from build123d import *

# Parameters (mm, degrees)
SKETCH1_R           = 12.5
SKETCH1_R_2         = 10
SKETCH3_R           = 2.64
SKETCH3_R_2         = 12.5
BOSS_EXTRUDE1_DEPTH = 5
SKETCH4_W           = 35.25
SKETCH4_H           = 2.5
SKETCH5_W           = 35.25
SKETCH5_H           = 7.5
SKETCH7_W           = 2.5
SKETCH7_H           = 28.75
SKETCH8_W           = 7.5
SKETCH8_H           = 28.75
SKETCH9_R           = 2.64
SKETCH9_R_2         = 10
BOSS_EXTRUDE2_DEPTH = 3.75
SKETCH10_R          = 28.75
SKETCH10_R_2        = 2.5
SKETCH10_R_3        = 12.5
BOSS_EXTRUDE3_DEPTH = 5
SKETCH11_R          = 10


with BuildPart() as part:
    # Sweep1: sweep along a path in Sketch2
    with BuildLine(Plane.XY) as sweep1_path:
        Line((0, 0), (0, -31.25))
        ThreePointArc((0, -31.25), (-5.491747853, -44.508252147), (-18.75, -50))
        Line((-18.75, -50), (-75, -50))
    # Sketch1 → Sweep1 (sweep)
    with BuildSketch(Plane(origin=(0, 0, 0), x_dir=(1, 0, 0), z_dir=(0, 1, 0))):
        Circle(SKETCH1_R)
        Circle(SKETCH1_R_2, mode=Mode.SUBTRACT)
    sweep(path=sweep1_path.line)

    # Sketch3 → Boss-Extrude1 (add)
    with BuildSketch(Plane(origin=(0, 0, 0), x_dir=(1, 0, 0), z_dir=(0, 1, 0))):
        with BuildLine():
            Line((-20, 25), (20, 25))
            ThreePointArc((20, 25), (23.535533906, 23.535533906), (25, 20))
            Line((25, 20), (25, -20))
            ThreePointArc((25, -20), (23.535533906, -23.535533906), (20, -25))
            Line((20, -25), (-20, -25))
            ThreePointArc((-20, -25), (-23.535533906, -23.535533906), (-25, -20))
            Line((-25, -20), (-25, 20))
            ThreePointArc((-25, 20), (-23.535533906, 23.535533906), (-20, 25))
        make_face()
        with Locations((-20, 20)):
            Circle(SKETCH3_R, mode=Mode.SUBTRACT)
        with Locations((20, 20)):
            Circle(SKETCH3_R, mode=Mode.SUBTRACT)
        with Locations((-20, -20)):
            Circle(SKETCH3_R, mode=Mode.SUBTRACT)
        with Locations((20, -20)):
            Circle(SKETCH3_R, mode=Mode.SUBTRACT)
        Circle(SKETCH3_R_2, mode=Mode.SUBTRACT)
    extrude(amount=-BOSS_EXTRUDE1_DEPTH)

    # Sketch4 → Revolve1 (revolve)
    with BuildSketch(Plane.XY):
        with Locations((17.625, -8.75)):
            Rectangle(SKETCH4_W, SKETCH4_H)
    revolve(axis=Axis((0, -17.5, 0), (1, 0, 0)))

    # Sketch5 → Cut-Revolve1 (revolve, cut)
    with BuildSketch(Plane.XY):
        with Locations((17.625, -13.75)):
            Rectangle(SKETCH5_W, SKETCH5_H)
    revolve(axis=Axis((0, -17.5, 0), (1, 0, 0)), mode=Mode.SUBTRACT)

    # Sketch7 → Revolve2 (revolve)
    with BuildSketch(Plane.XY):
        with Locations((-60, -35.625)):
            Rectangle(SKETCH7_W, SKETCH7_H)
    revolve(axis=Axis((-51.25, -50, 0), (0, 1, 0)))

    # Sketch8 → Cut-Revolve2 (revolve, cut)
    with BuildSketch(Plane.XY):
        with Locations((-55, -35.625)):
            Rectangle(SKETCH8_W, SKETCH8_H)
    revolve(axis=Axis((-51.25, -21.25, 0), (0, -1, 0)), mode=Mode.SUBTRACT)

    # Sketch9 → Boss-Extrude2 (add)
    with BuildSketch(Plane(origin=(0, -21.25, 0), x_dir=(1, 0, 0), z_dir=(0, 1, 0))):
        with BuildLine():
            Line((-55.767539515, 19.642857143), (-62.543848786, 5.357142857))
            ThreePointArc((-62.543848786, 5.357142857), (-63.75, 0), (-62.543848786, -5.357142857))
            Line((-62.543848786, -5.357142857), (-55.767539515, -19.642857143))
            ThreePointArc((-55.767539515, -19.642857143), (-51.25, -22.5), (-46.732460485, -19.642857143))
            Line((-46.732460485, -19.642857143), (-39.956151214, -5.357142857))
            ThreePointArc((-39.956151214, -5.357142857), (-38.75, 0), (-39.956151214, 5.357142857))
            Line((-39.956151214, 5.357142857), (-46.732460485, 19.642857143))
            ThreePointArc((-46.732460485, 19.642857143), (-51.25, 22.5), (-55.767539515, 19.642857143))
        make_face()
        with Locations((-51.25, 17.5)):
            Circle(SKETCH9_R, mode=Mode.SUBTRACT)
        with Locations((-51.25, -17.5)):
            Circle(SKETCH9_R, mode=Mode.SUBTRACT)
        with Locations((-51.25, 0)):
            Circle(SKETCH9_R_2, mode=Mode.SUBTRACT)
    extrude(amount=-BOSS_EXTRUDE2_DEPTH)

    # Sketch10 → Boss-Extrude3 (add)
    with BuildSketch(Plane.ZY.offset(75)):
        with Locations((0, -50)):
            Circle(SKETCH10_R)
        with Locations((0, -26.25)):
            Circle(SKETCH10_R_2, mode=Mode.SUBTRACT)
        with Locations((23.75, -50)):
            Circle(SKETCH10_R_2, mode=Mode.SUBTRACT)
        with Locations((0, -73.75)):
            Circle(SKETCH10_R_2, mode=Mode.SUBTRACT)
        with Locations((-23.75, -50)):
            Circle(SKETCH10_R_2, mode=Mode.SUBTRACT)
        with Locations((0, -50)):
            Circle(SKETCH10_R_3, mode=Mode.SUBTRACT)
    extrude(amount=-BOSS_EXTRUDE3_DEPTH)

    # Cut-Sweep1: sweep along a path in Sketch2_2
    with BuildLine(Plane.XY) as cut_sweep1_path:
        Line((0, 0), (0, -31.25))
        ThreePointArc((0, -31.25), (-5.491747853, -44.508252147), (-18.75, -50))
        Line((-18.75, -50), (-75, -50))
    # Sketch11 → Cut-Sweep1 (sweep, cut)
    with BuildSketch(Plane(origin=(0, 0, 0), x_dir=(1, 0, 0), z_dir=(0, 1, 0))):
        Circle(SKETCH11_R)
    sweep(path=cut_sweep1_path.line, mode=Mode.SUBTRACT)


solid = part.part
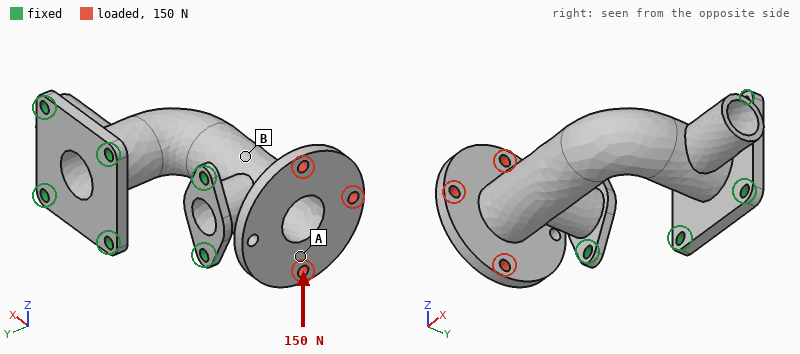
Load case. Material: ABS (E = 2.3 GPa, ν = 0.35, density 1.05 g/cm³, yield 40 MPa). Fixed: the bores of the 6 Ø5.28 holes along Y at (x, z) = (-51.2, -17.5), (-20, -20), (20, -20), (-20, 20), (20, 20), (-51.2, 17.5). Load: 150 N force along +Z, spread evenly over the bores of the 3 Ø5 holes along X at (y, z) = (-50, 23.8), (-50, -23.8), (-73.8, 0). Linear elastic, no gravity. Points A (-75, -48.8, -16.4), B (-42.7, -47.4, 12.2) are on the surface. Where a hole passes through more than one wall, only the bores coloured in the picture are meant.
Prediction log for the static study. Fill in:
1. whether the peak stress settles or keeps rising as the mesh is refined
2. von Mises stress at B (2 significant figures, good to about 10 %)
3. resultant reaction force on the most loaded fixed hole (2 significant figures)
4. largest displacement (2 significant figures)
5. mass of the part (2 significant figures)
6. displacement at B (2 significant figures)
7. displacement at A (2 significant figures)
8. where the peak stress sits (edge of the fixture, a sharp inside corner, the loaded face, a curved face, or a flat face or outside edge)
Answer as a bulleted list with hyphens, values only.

- keeps rising
- 2.3 MPa
- 170 N
- 0.97 mm
- 49 g
- 0.31 mm
- 0.56 mm
- edge of the fixture
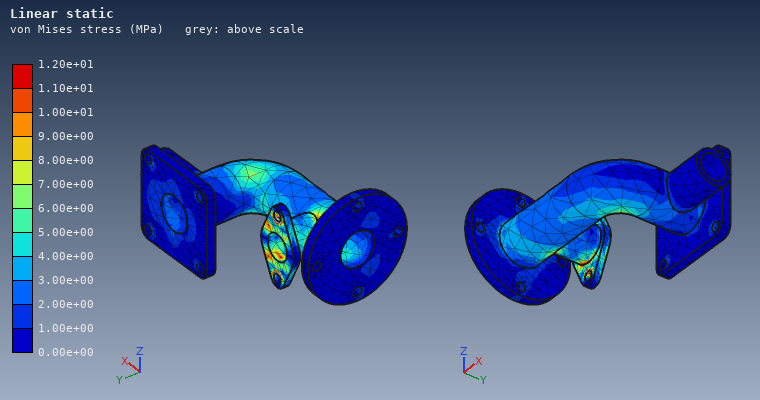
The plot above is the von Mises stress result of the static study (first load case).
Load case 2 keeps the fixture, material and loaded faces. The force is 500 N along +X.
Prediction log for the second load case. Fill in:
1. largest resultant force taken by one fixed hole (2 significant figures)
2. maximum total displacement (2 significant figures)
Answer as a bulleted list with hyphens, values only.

- 220 N
- 1.6 mm
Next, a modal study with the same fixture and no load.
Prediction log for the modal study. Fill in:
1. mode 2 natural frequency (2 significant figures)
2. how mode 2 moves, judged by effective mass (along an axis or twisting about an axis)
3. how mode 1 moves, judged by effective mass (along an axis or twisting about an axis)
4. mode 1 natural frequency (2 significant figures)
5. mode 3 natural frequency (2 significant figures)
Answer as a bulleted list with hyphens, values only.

- 790 Hz
- along X
- along Z
- 610 Hz
- 980 Hz
